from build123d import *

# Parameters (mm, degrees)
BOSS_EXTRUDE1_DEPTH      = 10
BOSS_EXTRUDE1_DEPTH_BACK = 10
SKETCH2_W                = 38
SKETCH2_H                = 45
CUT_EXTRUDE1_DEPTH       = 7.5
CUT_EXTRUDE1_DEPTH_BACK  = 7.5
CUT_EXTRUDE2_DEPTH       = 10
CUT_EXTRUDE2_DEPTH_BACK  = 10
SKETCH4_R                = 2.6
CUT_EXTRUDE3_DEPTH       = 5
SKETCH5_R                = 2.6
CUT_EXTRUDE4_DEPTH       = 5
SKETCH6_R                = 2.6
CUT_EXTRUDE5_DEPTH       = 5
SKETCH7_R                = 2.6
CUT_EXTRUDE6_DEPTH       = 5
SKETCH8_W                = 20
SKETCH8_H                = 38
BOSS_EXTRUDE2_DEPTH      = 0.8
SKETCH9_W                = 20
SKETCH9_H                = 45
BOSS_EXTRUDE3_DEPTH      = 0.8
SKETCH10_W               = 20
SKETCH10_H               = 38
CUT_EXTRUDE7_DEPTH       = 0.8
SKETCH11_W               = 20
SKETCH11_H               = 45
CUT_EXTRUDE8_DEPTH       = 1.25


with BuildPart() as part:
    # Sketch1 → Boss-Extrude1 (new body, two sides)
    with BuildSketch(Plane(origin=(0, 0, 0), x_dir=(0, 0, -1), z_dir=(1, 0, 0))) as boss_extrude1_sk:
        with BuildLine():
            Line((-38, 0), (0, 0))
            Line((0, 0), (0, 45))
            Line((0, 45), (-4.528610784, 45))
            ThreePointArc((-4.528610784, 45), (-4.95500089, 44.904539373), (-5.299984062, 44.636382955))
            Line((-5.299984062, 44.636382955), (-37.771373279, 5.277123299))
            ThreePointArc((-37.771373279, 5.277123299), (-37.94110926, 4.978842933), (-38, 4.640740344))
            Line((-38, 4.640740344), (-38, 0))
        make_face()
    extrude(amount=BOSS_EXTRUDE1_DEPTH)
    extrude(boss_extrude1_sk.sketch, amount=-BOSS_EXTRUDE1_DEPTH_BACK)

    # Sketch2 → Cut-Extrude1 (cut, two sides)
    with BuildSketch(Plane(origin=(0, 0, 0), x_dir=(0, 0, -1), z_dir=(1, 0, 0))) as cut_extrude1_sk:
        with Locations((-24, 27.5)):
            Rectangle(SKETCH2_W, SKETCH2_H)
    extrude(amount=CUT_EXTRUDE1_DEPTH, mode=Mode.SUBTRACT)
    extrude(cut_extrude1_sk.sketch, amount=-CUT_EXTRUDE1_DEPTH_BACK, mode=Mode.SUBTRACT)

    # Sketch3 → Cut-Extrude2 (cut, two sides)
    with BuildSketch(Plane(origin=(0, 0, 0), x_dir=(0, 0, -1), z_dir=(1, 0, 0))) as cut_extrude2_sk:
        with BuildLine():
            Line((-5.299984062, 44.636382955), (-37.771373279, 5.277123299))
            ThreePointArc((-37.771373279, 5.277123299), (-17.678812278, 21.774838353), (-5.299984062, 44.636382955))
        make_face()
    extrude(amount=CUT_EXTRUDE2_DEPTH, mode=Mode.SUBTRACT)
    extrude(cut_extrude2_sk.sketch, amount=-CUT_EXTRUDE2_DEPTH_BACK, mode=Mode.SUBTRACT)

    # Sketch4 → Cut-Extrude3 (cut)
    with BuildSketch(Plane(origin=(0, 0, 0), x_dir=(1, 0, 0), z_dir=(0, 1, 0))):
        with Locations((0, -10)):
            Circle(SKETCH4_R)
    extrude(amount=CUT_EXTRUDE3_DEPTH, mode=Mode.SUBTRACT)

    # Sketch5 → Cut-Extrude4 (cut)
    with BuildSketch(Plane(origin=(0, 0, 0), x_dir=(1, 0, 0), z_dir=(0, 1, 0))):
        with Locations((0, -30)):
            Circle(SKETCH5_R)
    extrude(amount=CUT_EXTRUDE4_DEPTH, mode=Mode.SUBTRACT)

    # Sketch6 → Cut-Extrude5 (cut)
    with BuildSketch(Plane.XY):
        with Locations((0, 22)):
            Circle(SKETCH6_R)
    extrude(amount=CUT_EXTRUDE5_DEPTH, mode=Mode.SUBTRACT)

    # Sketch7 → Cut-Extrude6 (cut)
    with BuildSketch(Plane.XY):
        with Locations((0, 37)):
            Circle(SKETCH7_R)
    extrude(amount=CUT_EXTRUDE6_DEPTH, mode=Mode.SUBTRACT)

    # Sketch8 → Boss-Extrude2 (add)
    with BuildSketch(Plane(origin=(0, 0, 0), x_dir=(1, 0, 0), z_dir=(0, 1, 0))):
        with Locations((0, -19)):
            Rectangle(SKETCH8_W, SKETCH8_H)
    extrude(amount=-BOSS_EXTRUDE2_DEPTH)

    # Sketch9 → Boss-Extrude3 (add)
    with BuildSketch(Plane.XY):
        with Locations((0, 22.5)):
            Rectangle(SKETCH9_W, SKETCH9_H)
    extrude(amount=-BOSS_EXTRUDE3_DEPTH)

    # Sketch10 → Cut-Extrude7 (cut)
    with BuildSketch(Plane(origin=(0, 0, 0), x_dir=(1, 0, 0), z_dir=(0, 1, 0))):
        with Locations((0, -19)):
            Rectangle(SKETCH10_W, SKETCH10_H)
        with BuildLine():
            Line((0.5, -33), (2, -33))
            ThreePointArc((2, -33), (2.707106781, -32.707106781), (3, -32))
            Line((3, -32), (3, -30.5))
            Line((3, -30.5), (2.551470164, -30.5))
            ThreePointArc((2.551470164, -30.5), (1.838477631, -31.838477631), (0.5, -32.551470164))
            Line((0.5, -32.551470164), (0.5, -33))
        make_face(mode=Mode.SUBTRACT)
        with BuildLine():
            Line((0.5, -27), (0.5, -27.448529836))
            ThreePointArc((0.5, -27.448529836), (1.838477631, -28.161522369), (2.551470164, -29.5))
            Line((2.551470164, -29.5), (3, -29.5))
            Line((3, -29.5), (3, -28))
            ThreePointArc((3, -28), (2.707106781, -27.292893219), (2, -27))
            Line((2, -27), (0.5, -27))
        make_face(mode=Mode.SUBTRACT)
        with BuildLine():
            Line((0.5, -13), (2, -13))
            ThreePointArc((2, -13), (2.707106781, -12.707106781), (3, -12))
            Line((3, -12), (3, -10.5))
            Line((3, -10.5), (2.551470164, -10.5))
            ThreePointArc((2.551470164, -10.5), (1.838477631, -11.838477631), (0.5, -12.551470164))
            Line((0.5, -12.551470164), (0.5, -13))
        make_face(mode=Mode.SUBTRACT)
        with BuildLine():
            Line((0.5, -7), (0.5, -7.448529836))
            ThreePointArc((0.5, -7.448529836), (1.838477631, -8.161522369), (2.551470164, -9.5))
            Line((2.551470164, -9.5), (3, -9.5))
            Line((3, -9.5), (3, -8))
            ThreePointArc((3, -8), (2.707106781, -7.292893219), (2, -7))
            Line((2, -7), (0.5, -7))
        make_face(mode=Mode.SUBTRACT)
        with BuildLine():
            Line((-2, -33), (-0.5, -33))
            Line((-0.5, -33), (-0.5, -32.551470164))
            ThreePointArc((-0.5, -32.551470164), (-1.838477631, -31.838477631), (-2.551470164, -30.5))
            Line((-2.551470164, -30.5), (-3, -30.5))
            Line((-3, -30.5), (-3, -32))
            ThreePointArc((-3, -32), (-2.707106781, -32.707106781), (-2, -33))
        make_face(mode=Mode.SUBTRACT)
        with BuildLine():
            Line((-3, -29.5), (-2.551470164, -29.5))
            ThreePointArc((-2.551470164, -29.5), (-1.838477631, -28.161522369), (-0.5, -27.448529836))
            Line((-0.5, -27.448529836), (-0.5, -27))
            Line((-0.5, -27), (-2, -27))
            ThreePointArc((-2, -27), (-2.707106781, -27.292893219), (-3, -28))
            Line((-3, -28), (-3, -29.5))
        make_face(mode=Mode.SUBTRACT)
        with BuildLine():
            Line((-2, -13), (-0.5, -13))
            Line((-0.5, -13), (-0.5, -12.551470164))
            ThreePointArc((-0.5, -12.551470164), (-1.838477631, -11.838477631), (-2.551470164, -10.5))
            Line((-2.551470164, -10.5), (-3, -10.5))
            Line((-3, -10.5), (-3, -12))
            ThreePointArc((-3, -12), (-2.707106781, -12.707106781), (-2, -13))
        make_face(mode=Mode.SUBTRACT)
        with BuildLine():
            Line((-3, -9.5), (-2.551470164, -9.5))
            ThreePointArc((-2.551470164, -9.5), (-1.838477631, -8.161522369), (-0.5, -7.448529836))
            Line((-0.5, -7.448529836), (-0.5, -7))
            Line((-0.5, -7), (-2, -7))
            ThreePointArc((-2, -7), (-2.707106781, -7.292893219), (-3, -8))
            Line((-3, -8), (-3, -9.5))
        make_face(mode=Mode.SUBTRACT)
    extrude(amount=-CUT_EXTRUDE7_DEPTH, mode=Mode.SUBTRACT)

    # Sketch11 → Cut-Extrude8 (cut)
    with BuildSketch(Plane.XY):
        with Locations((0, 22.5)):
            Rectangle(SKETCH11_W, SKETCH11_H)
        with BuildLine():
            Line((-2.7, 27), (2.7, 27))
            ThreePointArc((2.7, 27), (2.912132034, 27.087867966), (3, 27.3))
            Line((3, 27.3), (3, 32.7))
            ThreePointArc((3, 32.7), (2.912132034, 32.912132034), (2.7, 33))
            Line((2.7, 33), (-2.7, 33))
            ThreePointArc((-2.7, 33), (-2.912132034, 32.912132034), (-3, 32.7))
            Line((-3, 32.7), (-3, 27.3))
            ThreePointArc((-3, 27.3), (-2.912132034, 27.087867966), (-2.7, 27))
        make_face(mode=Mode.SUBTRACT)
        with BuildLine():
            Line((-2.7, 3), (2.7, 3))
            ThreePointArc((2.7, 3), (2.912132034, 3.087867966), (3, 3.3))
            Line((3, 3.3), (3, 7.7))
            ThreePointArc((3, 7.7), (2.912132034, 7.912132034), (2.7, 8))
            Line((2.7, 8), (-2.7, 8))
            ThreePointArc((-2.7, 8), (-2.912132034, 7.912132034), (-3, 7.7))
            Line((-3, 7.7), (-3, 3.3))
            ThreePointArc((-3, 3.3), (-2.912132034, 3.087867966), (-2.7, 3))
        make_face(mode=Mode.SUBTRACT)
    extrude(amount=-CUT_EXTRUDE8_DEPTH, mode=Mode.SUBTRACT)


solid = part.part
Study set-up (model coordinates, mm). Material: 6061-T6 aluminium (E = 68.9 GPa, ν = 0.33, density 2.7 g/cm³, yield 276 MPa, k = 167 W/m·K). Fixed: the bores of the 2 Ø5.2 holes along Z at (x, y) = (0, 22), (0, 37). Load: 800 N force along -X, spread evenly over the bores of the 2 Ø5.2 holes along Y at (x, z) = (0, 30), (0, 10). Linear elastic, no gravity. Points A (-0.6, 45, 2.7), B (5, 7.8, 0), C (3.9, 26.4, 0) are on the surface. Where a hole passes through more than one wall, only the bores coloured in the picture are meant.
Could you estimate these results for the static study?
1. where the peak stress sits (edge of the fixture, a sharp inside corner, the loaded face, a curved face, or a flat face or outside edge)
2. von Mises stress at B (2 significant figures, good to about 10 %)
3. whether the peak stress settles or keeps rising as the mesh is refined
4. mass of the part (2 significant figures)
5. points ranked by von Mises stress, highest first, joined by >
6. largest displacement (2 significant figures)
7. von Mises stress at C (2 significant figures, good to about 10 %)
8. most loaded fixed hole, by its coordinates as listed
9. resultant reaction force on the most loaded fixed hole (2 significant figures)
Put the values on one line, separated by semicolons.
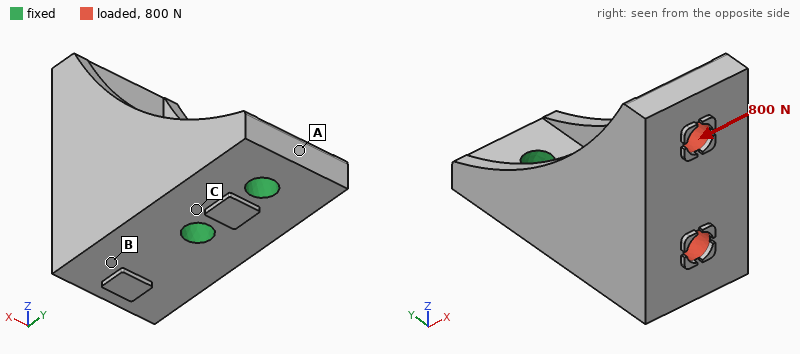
edge of the fixture; 29 MPa; keeps rising; 27 g; C > B > A; 0.22 mm; 46 MPa; (0, 22); 1.4 kN
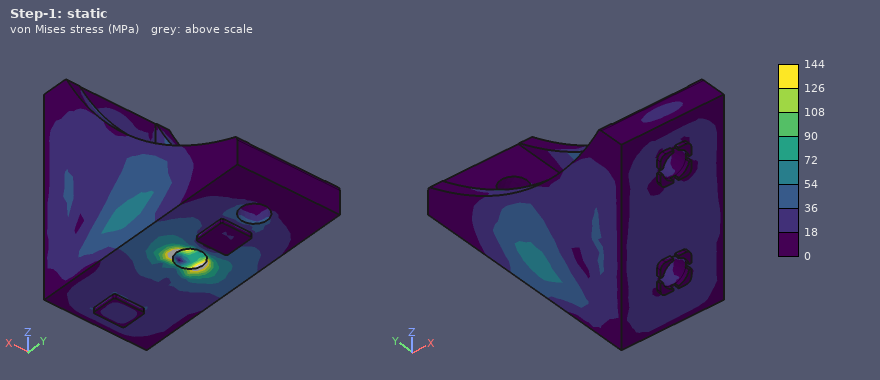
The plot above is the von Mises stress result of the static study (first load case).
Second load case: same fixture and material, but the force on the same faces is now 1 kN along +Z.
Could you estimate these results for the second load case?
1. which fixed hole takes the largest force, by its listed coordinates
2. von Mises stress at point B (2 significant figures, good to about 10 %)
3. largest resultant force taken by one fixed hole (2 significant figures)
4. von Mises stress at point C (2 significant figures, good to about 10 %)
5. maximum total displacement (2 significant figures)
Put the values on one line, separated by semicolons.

(0, 22); 11 MPa; 1.7 kN; 23 MPa; 89 µm
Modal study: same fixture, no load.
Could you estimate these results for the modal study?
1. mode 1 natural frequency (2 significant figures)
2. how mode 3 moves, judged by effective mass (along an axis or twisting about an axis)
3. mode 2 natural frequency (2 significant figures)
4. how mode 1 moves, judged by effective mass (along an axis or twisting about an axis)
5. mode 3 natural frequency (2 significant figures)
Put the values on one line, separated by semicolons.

3200 Hz; along X; 4900 Hz; along X; 12 kHz
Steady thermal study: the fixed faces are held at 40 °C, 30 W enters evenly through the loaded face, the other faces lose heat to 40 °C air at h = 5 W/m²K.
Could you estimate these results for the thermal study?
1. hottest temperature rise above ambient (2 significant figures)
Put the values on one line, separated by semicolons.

38 K
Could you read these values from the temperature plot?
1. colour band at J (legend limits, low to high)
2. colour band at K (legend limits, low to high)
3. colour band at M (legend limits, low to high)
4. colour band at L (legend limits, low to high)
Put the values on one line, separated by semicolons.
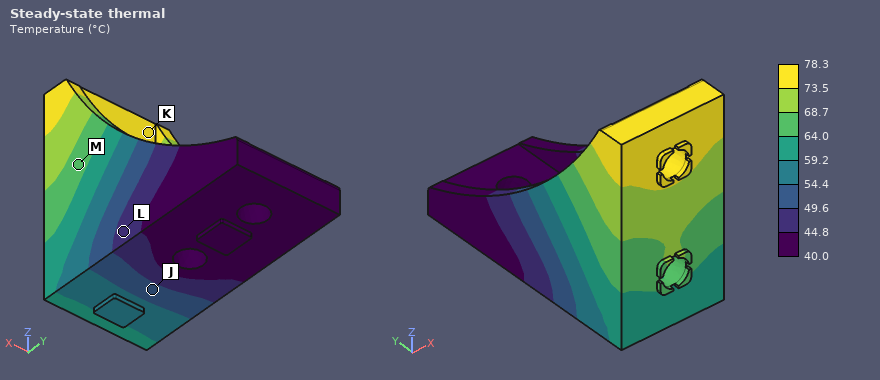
49.6 to 54.4 °C; 73.5 to 78.3 °C; 64.0 to 68.7 °C; 44.8 to 49.6 °C
